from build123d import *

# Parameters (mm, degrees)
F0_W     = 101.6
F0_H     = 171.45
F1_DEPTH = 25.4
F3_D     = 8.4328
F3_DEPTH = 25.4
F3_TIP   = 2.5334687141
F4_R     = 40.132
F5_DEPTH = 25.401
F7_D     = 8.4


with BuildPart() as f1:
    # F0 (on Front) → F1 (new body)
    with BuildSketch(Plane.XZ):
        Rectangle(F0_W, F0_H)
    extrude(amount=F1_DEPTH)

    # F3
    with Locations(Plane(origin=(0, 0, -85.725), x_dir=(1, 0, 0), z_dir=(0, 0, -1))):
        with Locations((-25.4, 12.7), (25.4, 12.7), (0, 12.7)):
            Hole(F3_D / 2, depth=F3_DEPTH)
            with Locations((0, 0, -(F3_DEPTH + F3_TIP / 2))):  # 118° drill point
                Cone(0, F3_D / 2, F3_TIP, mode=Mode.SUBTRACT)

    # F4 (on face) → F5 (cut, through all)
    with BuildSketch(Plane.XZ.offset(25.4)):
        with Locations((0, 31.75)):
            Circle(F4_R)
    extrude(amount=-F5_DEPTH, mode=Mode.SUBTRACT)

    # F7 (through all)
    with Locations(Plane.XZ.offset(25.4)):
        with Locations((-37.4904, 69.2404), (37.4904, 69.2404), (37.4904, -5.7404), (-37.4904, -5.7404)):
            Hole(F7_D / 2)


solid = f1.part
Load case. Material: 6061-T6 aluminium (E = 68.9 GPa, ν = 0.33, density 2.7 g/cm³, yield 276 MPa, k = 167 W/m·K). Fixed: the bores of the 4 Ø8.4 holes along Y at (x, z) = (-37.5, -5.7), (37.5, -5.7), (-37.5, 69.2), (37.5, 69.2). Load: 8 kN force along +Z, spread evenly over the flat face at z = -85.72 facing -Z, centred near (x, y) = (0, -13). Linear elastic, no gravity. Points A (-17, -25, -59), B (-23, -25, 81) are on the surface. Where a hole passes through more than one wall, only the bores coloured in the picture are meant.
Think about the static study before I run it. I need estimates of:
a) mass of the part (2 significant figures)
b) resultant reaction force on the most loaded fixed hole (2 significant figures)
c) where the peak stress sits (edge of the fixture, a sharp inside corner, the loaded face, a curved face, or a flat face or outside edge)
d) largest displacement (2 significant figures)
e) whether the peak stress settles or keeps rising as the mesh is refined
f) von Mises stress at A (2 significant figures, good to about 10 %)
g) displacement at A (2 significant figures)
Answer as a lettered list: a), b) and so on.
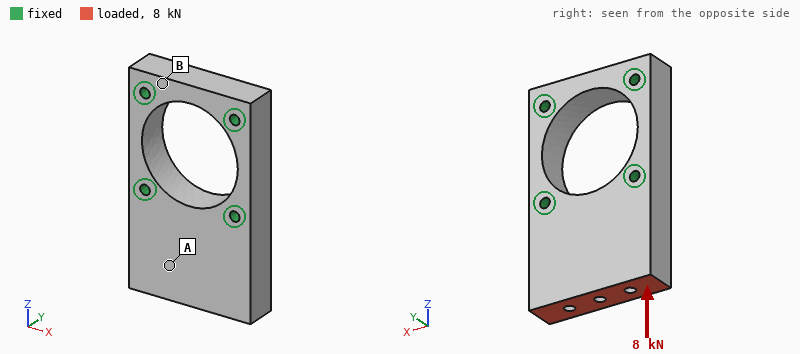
a) 820 g
b) 4.1 kN
c) edge of the fixture
d) 4.8 µm
e) keeps rising
f) 2.9 MPa
g) 3.5 µm
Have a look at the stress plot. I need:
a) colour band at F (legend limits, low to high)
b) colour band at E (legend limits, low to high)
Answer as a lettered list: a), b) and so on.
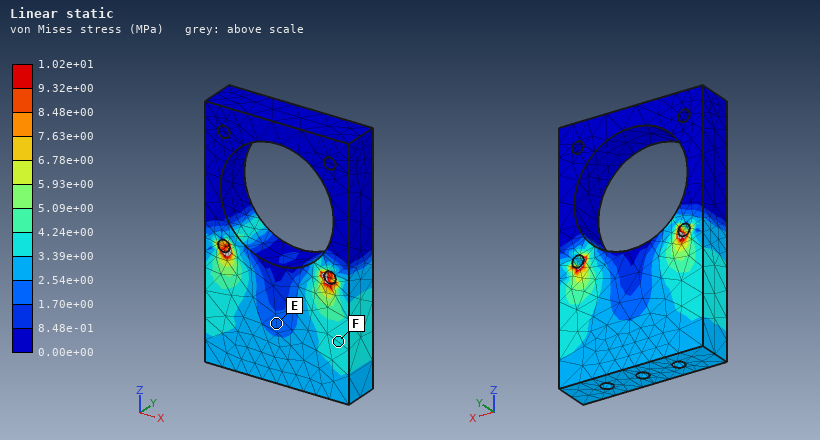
a) 3.39e+00 to 4.24e+00 MPa
b) 1.70e+00 to 2.54e+00 MPa
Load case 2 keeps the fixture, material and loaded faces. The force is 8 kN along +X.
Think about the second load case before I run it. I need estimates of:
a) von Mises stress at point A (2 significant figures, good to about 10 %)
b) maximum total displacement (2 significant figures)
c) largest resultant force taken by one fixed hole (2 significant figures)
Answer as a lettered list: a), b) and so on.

a) 8.2 MPa
b) 27 µm
c) 8.7 kN
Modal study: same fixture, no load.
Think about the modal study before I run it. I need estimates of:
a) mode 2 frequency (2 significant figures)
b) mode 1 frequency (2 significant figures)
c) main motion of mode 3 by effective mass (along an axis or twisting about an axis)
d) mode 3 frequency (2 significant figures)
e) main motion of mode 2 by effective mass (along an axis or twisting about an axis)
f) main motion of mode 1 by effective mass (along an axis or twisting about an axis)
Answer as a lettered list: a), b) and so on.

a) 5300 Hz
b) 2500 Hz
c) along X
d) 6900 Hz
e) twisting about Z
f) along Y
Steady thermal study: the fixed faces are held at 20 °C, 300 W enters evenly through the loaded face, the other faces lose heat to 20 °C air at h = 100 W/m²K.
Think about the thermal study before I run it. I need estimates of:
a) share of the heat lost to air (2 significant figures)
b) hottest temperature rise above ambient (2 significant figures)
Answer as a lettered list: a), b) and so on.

a) 23 %
b) 54 K
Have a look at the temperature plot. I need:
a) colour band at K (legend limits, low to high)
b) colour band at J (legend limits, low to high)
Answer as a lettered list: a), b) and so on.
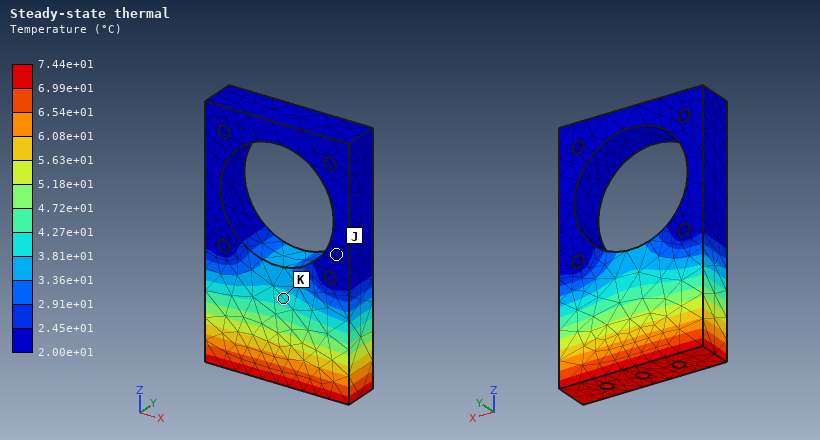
a) 3.81e+01 to 4.27e+01 °C
b) 2.00e+01 to 2.45e+01 °C
